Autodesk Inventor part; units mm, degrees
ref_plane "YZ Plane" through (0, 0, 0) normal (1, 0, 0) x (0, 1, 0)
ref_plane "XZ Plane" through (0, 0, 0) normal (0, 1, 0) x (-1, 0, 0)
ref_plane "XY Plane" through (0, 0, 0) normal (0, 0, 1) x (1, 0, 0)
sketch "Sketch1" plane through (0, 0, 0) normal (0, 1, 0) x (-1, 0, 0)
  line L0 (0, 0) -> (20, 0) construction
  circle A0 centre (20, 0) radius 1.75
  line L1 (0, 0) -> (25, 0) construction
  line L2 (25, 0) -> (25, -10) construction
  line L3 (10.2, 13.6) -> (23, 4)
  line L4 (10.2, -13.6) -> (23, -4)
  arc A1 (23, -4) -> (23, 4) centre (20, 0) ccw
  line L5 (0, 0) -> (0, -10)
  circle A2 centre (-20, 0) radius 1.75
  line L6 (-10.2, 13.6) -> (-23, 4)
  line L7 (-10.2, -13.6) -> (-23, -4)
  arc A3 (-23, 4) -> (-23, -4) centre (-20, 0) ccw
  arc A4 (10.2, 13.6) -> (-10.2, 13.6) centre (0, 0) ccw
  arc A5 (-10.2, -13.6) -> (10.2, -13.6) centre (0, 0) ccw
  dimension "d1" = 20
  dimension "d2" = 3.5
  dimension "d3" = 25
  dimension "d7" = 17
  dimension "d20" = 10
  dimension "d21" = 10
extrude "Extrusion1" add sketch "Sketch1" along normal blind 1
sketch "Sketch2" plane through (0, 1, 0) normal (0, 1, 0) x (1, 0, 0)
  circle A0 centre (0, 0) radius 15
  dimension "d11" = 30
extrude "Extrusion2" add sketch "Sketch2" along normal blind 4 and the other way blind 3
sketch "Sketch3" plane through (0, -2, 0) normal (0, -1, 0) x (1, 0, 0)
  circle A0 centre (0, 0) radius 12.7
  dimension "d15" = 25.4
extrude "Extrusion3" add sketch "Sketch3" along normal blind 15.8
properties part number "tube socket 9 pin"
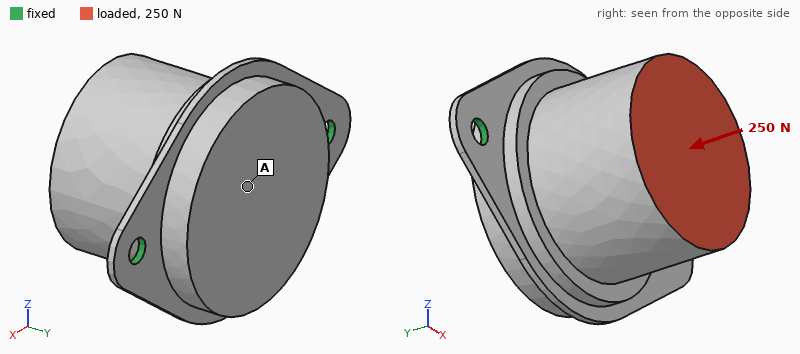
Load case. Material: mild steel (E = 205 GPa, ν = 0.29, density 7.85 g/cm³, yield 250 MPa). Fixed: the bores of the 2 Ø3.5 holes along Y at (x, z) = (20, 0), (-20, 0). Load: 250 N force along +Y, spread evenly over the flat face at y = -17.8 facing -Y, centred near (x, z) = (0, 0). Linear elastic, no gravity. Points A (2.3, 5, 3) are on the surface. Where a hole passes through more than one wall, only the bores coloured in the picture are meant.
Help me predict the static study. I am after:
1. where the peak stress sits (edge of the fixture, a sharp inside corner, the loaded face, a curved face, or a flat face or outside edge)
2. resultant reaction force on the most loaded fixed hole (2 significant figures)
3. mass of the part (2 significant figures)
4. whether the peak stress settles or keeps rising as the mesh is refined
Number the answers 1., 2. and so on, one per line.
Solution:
1. edge of the fixture
2. 130 N
3. 100 g
4. keeps rising
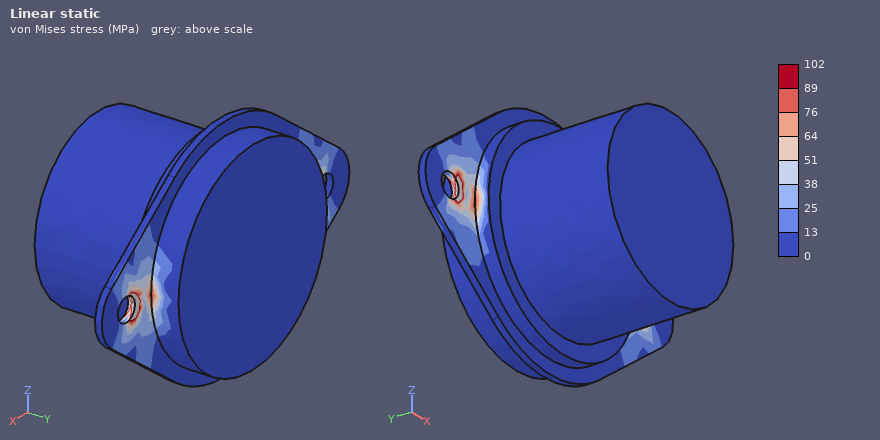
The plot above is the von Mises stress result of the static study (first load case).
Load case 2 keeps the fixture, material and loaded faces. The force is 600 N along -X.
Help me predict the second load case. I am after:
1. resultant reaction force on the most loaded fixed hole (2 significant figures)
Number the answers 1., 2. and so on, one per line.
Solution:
1. 440 N
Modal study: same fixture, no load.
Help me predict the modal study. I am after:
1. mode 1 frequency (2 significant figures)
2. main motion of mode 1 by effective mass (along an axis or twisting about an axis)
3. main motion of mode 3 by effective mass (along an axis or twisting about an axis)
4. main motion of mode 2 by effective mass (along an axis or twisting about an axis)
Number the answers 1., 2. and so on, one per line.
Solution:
1. 780 Hz
2. along Z
3. along X
4. along Y
